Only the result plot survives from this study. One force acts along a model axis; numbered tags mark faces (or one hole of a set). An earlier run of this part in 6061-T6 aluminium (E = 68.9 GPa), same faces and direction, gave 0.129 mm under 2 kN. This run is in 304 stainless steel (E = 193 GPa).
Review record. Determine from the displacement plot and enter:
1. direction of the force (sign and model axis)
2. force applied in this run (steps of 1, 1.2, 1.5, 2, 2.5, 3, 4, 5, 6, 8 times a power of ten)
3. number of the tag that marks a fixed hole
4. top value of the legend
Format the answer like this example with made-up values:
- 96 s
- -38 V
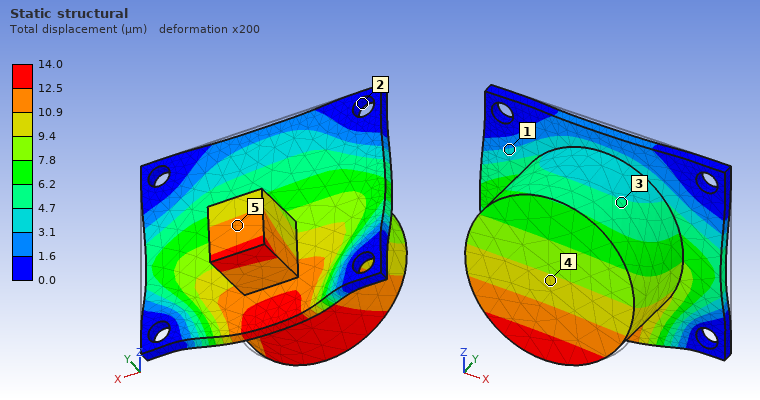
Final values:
- -Y
- 600 N
- 2
- 14.0 µm
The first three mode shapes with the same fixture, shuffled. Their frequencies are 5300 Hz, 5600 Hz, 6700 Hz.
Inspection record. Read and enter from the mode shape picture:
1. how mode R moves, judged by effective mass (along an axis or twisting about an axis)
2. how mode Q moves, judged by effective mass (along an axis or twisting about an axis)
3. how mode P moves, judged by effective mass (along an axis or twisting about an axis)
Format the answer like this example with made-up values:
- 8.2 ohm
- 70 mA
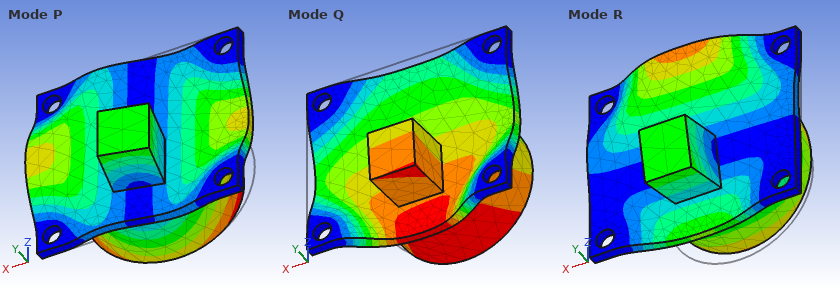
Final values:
- along Z
- along Y
- along X
